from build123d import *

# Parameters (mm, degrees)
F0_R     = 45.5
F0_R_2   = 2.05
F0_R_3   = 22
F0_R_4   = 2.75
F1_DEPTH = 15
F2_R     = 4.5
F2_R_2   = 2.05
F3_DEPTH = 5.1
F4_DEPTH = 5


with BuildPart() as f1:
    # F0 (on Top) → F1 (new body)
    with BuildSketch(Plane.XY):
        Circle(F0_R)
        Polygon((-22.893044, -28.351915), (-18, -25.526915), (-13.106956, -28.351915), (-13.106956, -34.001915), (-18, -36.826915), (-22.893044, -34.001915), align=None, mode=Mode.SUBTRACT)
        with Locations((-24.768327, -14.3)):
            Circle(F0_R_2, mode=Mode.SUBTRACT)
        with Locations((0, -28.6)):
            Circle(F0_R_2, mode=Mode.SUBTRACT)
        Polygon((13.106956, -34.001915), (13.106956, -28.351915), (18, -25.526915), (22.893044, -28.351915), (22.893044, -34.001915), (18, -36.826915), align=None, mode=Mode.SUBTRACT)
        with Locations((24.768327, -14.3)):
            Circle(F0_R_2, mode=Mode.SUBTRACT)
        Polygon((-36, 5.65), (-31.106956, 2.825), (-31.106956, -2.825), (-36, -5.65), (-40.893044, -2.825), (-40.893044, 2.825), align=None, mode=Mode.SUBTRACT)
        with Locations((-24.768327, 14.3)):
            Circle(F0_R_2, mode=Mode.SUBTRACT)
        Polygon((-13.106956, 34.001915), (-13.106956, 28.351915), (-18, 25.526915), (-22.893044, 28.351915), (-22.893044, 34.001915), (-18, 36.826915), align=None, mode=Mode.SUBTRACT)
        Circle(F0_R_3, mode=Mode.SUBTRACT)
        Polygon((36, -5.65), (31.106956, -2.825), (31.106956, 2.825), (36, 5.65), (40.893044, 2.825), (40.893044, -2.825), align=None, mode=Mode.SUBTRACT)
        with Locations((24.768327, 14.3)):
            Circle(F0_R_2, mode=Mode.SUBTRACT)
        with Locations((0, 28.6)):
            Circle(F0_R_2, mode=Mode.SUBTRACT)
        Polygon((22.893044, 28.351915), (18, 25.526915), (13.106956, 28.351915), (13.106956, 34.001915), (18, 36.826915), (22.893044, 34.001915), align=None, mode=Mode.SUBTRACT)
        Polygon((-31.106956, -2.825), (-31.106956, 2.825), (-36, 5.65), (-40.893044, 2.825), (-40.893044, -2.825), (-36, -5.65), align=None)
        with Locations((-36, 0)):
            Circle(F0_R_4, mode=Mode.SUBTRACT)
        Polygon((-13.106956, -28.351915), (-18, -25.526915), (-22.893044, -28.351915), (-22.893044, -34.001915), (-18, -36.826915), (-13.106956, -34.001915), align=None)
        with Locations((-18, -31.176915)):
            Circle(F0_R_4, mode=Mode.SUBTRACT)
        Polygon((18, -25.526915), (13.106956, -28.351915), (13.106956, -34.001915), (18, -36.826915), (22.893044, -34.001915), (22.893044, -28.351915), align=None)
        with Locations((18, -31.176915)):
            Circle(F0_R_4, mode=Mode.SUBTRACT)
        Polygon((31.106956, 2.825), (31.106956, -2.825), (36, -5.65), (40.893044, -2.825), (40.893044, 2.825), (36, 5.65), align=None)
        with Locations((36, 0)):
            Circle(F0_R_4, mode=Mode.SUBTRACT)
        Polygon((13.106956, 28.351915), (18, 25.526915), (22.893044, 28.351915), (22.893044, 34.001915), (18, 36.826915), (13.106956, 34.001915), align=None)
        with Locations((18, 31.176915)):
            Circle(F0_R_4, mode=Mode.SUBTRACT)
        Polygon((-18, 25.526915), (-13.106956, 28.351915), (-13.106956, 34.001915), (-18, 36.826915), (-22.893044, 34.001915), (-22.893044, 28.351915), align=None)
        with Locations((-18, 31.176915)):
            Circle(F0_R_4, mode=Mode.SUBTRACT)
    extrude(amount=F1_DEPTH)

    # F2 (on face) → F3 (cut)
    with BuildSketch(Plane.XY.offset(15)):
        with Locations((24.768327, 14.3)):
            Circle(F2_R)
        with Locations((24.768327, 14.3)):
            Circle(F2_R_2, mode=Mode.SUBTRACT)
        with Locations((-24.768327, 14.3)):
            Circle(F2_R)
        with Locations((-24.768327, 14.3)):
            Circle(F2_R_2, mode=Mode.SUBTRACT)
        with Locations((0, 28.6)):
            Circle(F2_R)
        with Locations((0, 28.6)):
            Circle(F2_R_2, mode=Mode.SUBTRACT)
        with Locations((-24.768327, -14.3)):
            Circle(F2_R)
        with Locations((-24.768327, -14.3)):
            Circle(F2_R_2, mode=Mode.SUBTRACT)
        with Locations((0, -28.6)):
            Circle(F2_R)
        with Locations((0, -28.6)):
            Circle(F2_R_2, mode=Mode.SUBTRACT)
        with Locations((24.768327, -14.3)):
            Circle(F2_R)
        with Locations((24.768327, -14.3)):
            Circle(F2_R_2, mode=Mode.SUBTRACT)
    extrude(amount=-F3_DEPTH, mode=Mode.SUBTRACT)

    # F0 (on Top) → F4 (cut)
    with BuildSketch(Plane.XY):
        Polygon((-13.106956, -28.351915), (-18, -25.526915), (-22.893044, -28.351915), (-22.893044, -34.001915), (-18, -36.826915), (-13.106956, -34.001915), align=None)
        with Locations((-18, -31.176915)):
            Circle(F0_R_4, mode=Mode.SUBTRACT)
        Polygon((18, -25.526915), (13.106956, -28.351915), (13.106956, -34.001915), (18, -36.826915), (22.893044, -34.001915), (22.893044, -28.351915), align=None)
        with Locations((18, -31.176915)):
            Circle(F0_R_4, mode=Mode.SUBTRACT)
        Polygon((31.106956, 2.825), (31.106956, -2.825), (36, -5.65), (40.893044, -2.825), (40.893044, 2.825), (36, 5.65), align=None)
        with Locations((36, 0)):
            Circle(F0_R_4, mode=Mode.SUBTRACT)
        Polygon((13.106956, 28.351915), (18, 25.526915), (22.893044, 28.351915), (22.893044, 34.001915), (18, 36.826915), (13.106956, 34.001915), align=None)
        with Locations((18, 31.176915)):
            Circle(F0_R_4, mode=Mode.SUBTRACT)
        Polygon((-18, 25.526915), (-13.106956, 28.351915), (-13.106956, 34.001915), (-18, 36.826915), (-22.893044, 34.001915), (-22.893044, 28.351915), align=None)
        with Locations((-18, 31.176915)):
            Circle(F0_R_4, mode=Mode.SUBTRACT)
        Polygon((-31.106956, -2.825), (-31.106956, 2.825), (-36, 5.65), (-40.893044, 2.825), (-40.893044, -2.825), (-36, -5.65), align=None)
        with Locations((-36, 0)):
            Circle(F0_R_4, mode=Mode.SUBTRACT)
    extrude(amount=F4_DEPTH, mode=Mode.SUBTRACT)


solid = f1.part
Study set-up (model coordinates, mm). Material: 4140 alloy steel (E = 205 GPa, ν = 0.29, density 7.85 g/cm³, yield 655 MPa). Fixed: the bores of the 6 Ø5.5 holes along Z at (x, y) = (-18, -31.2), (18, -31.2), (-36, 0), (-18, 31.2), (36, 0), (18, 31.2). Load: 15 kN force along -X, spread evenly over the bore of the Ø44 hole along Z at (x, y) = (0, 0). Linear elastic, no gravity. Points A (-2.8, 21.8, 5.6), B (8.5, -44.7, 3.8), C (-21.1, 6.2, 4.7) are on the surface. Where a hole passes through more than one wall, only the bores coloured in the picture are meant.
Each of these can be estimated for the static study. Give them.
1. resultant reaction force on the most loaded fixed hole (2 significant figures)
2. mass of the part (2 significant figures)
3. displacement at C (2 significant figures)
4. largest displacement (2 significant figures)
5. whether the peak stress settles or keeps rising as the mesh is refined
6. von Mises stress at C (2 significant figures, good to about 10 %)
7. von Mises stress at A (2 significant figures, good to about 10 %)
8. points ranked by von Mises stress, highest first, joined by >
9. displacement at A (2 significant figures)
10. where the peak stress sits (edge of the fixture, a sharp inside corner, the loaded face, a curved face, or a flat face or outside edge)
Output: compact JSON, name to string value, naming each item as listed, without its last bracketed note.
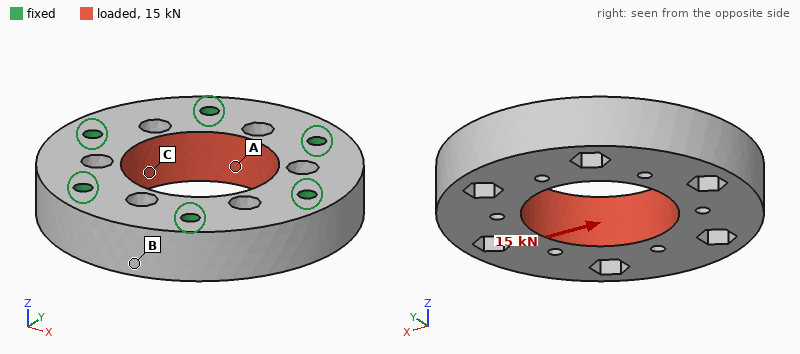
{"resultant reaction force on the most loaded fixed hole": "3.0 kN", "mass of the part": "530 g", "displacement at C": "1.4 µm", "largest displacement": "1.8 µm", "whether the peak stress settles or keeps rising as the mesh is refined": "keeps rising", "von Mises stress at C": "9.2 MPa", "von Mises stress at A": "14 MPa", "points ranked by von Mises stress, highest first, joined by >": "A > C > B", "displacement at A": "1.1 µm", "where the peak stress sits": "edge of the fixture"}
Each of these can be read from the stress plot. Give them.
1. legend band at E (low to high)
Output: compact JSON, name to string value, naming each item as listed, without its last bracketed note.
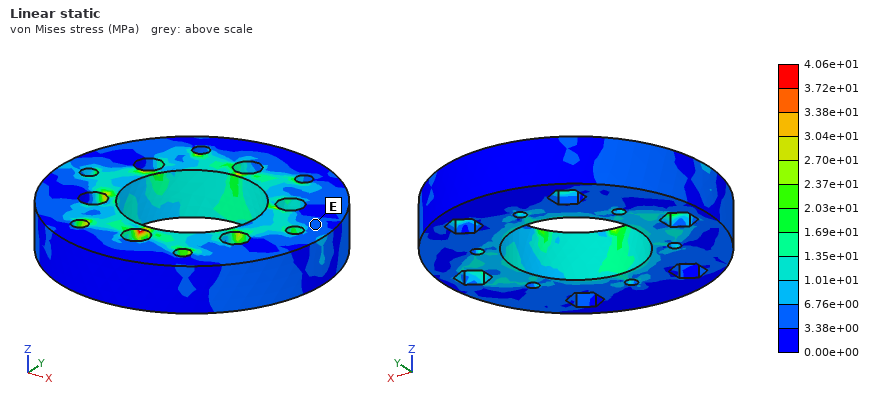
{"legend band at E": "3.38e+00 to 6.76e+00 MPa"}
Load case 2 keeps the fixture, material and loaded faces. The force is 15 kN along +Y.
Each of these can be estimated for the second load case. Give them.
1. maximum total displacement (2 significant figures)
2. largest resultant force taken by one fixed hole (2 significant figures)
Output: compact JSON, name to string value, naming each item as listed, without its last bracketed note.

{"maximum total displacement": "2.0 µm", "largest resultant force taken by one fixed hole": "2.8 kN"}
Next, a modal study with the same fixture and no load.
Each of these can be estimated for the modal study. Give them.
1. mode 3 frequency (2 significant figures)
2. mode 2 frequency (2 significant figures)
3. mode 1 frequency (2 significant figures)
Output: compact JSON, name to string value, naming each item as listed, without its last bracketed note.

{"mode 3 frequency": "23 kHz", "mode 2 frequency": "23 kHz", "mode 1 frequency": "23 kHz"}
